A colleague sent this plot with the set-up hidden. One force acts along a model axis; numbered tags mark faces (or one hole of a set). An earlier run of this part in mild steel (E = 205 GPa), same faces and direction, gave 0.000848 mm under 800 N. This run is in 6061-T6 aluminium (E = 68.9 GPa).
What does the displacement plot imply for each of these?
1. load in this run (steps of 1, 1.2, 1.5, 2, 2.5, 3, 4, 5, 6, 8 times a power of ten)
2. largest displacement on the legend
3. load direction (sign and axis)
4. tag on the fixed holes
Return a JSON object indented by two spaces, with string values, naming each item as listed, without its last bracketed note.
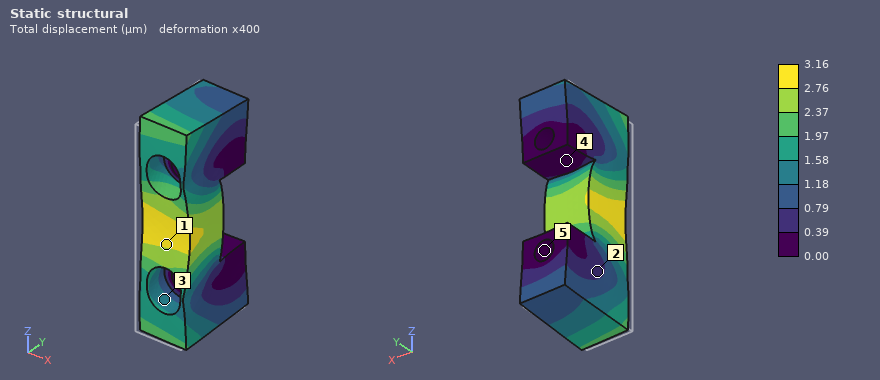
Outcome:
{
  "load in this run": "1 kN",
  "largest displacement on the legend": "3.16 µm",
  "load direction": "+Y",
  "tag on the fixed holes": "5"
}
